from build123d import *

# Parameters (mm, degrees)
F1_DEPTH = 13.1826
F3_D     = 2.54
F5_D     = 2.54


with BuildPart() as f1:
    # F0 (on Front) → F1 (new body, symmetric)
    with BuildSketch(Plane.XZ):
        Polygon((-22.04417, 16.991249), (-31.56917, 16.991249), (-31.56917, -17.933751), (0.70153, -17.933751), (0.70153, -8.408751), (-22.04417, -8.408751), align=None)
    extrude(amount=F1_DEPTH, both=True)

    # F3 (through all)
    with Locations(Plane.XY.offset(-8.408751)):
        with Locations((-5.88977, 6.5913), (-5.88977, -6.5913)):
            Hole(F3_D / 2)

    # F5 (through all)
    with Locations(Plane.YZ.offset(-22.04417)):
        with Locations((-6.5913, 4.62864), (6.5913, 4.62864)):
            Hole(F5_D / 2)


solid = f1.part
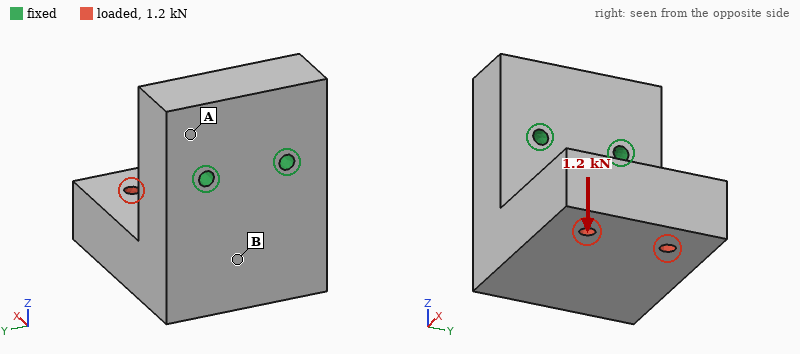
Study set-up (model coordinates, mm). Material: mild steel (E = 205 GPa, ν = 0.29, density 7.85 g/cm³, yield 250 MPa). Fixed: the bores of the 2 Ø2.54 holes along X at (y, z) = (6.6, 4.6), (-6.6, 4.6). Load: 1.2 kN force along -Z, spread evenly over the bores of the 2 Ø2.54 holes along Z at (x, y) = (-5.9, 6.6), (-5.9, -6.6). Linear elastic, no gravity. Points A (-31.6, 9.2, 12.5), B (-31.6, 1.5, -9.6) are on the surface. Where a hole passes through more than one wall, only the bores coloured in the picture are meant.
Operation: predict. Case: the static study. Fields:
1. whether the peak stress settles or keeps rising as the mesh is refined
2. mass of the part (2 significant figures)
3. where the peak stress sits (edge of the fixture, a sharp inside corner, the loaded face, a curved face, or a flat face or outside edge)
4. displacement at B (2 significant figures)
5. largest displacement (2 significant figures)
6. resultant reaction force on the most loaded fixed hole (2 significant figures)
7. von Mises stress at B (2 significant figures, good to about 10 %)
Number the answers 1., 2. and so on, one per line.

1. keeps rising
2. 110 g
3. edge of the fixture
4. 9.3 µm
5. 47 µm
6. 610 N
7. 38 MPa
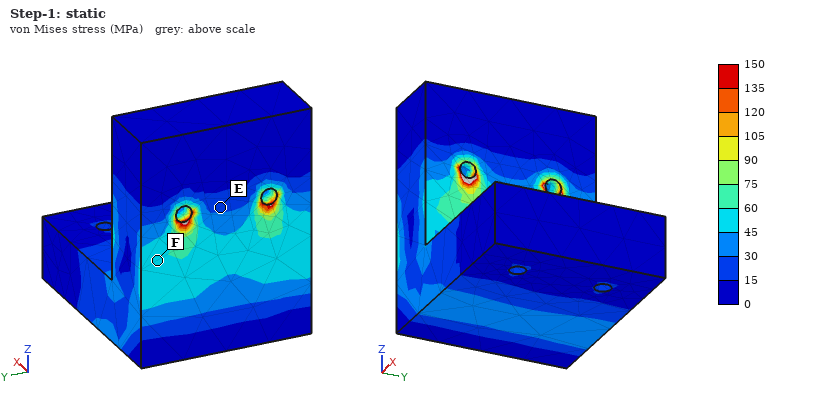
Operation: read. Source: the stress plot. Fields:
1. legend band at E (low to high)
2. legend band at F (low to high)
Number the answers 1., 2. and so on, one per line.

1. 15 to 30 MPa
2. 45 to 60 MPa
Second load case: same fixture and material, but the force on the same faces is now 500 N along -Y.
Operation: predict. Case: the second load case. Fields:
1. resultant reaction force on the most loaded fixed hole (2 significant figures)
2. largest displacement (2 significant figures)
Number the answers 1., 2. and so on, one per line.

1. 830 N
2. 9.4 µm
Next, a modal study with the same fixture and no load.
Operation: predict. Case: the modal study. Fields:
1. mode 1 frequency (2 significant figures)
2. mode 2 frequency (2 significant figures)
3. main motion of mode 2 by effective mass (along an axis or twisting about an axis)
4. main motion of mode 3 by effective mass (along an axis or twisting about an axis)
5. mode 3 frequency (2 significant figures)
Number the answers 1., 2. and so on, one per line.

1. 4700 Hz
2. 7000 Hz
3. along Y
4. along X
5. 13 kHz
